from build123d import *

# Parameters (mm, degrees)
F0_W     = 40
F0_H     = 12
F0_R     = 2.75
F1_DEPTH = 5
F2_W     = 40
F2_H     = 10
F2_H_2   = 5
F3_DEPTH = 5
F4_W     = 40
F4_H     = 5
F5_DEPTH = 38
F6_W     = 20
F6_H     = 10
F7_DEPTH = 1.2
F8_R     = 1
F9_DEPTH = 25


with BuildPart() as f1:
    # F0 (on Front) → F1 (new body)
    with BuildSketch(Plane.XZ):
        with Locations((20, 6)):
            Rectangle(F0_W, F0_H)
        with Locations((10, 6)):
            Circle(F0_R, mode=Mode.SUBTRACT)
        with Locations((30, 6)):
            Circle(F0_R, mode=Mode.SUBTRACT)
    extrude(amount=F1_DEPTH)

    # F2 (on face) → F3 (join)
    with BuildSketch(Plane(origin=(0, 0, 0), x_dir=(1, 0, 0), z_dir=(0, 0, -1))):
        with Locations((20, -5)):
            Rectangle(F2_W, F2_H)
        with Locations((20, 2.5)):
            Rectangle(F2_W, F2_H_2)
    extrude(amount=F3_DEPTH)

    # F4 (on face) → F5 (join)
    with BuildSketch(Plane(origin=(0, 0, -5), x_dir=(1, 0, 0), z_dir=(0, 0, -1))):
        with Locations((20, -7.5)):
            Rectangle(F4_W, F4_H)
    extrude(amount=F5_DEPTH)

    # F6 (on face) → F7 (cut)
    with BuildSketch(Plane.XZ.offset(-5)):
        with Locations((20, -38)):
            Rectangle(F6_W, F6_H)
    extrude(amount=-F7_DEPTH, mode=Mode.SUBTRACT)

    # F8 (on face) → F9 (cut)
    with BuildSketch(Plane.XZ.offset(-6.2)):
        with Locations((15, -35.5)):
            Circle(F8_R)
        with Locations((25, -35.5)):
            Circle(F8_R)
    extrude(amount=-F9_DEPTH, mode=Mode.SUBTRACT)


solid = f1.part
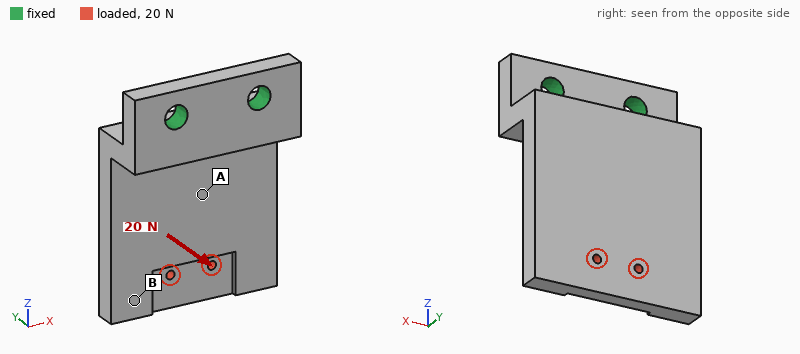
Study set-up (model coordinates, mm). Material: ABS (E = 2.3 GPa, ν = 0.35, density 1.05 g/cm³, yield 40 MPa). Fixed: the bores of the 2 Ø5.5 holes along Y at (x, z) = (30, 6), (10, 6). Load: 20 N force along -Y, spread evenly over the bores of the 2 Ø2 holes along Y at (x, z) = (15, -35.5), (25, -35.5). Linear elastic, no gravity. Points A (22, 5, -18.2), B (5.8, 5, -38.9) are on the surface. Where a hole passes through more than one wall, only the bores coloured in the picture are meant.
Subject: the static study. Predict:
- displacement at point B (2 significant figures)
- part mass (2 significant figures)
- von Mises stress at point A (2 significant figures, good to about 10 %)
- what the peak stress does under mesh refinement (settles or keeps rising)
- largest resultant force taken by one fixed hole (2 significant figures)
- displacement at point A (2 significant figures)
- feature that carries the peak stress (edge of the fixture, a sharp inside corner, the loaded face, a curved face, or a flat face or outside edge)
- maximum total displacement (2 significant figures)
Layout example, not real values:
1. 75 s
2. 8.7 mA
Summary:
1. 0.65 mm
2. 13 g
3. 2.0 MPa
4. keeps rising
5. 10 N
6. 0.25 mm
7. edge of the fixture
8. 0.76 mm
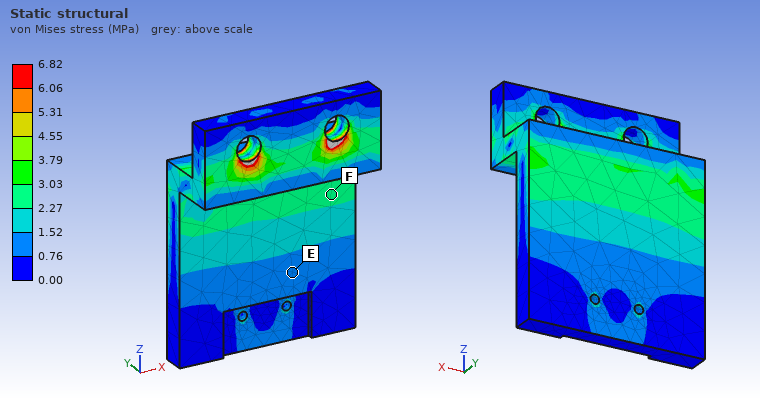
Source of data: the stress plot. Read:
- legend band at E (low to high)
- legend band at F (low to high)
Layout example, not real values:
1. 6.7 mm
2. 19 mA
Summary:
1. 0.76 to 1.52 MPa
2. 2.27 to 3.03 MPa
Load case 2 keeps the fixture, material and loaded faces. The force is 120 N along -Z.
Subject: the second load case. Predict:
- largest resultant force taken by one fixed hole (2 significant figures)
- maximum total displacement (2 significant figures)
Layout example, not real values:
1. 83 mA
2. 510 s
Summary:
1. 60 N
2. 0.68 mm
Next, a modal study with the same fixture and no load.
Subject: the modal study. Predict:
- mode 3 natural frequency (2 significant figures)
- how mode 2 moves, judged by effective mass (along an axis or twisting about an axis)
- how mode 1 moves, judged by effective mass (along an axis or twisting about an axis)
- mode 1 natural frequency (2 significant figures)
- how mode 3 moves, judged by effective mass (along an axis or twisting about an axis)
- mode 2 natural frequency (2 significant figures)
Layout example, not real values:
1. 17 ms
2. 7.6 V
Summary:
1. 1800 Hz
2. along X
3. along Y
4. 470 Hz
5. along X
6. 1200 Hz
